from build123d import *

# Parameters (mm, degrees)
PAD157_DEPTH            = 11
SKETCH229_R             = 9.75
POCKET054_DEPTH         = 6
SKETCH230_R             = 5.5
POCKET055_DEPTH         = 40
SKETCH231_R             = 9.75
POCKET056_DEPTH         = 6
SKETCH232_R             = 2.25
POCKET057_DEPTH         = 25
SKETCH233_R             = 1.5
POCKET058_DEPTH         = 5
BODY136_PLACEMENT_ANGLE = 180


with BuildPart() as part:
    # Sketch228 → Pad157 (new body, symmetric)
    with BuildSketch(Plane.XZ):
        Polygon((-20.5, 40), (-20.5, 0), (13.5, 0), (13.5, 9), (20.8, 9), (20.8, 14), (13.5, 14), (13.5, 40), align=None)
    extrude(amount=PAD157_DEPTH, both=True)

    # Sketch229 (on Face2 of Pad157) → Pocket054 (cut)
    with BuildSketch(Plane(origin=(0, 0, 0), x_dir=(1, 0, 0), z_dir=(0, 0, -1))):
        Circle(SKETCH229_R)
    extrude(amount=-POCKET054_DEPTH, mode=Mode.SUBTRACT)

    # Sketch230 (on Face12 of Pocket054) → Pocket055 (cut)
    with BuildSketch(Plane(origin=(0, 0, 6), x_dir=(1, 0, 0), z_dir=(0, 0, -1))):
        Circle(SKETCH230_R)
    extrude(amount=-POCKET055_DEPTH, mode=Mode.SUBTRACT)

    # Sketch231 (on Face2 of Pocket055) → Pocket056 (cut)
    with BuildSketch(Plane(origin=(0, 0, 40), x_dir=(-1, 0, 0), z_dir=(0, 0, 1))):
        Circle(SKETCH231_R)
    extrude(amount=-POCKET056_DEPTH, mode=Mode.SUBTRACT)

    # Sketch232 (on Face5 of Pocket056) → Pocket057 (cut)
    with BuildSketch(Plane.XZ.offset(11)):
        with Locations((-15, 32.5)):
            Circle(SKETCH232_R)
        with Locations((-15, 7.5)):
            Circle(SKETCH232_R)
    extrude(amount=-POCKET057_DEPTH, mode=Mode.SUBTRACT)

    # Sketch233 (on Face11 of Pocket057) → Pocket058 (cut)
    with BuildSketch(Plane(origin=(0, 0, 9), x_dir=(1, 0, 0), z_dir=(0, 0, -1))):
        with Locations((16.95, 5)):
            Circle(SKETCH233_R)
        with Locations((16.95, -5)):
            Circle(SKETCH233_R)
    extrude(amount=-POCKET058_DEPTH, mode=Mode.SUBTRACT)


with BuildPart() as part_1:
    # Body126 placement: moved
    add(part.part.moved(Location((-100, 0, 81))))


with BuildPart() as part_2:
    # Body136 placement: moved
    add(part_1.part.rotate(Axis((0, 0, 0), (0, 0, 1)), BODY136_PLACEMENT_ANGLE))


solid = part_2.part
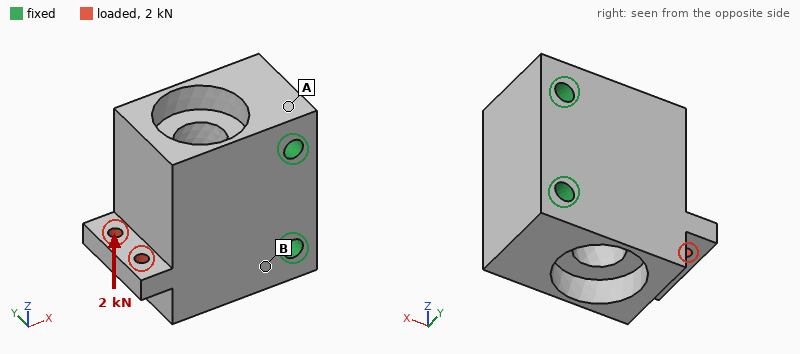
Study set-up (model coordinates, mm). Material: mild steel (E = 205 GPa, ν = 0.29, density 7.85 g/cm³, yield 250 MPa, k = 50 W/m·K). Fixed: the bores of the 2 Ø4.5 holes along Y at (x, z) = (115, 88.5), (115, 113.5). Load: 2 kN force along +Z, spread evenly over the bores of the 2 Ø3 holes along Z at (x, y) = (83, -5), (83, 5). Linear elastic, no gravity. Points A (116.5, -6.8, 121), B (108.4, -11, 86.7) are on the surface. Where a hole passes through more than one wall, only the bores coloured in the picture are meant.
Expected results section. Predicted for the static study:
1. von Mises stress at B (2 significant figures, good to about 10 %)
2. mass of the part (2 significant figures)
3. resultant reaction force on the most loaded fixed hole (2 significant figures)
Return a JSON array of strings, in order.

["20 MPa", "190 g", "2.6 kN"]
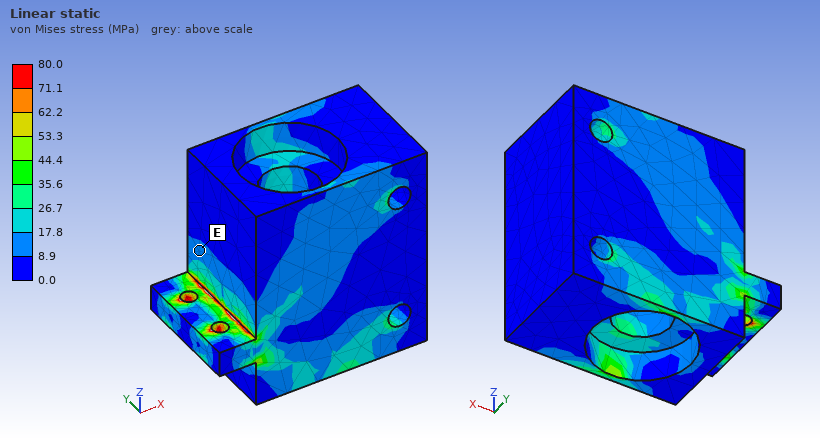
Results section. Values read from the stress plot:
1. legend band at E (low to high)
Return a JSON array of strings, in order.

["8.9 to 17.8 MPa"]
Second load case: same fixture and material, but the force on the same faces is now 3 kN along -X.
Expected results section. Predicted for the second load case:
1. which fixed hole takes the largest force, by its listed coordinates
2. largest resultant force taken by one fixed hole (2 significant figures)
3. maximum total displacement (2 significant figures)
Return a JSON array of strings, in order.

["(115, 88.5)", "2.5 kN", "4.1 µm"]
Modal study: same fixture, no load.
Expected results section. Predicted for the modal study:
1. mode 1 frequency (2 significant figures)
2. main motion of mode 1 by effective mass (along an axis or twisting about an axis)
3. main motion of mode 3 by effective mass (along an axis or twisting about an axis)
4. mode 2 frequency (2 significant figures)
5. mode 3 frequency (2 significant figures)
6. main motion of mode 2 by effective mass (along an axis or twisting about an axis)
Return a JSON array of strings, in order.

["11 kHz", "along Y", "twisting about X", "16 kHz", "18 kHz", "along Z"]
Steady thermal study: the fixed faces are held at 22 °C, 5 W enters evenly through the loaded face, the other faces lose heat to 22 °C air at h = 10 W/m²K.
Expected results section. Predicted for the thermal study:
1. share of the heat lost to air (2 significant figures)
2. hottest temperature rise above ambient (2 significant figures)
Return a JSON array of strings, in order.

["4.6 %", "13 K"]
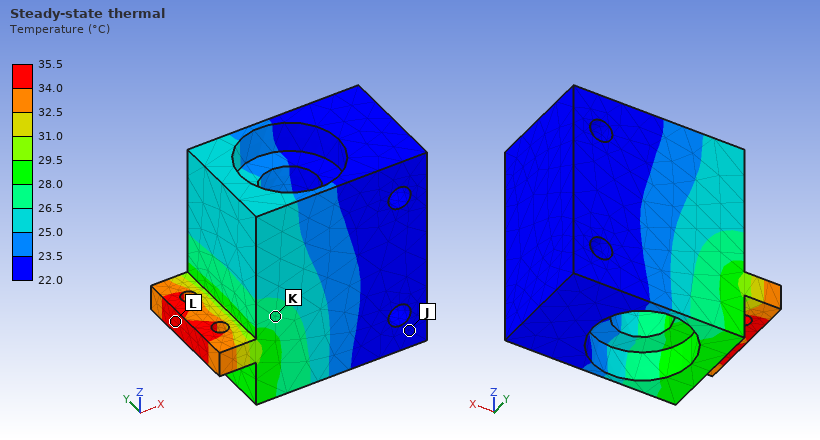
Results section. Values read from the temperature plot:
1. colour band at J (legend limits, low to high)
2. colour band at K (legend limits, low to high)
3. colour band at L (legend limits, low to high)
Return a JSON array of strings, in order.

["22.0 to 23.5 °C", "26.5 to 28.0 °C", "34.0 to 35.5 °C"]
